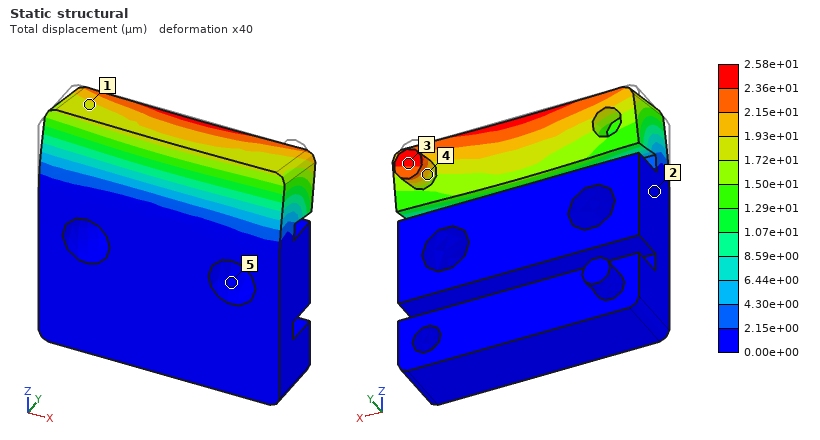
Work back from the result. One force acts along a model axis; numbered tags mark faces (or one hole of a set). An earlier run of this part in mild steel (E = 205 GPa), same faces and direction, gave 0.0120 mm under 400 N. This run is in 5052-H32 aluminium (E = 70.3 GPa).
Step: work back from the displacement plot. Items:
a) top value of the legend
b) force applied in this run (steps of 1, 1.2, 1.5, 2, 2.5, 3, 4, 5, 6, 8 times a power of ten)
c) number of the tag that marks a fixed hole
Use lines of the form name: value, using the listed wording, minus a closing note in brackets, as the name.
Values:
top value of the legend: 2.58e+01 µm
force applied in this run: 300 N
number of the tag that marks a fixed hole: 5
